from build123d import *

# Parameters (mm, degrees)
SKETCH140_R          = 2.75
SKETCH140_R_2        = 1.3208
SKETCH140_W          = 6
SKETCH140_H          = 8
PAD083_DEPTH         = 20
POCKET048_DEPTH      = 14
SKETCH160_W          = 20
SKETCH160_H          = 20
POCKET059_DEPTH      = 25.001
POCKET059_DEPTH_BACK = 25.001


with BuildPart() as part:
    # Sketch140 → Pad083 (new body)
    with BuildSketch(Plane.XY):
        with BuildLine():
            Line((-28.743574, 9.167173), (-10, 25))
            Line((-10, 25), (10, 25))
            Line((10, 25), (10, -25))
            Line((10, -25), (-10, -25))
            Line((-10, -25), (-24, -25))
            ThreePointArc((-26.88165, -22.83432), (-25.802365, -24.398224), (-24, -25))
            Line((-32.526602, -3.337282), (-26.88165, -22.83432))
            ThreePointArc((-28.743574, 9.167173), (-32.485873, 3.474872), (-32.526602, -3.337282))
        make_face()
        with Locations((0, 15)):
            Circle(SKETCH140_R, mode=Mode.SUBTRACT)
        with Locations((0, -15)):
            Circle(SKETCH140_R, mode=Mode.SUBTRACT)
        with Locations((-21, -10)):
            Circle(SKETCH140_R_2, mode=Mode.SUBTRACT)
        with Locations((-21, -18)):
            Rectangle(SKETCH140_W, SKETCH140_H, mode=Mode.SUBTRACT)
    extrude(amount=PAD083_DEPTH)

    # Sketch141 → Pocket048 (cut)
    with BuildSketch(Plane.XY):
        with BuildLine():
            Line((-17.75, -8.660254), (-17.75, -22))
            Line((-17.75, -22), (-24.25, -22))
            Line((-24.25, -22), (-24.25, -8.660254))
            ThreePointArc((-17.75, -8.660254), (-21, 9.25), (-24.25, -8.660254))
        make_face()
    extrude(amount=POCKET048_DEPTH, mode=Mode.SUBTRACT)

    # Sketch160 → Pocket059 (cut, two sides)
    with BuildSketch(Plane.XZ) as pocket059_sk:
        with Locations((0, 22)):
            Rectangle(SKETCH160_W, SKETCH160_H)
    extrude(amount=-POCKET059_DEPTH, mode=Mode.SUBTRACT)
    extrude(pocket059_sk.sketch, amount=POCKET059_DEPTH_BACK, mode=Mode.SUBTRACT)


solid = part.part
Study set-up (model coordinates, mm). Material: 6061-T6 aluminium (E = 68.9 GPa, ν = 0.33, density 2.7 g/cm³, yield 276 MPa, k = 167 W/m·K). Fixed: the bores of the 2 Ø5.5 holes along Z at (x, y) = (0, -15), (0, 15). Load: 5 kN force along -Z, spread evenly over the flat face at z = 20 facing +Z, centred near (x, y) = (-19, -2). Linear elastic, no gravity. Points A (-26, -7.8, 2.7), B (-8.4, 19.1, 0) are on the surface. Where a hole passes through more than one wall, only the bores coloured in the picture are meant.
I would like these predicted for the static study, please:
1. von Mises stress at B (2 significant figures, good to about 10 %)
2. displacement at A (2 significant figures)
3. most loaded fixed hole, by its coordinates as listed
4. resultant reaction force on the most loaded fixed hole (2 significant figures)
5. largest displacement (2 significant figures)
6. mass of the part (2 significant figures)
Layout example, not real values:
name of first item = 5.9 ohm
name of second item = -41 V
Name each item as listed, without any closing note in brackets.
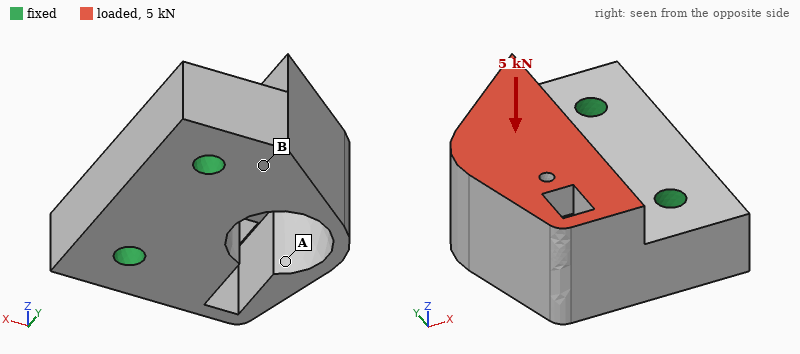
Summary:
von Mises stress at B = 58 MPa
displacement at A = 0.075 mm
most loaded fixed hole, by its coordinates as listed = (0, -15)
resultant reaction force on the most loaded fixed hole = 2.7 kN
largest displacement = 0.10 mm
mass of the part = 62 g
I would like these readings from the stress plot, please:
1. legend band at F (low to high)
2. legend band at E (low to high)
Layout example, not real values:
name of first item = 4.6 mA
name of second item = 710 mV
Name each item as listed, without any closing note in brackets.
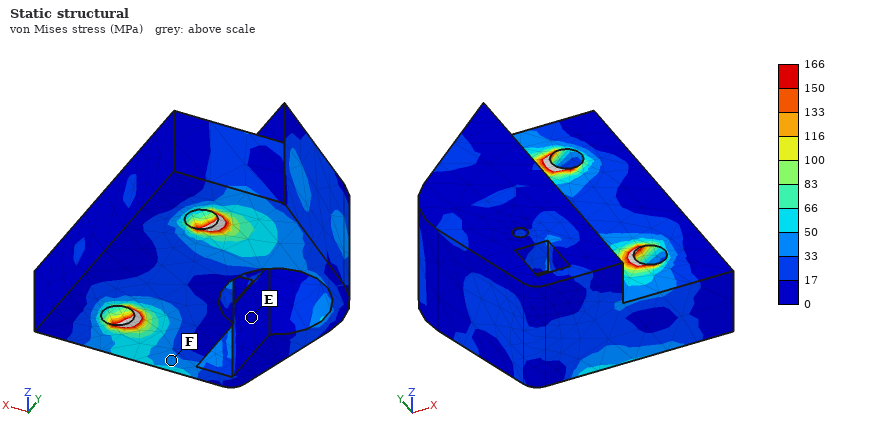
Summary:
legend band at F = 33 to 50 MPa
legend band at E = 0 to 17 MPa
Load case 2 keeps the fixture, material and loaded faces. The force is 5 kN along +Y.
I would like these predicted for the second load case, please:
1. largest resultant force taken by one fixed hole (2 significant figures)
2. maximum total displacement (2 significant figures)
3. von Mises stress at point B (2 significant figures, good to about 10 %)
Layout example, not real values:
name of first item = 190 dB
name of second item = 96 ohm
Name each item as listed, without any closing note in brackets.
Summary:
largest resultant force taken by one fixed hole = 4.1 kN
maximum total displacement = 33 µm
von Mises stress at point B = 12 MPa
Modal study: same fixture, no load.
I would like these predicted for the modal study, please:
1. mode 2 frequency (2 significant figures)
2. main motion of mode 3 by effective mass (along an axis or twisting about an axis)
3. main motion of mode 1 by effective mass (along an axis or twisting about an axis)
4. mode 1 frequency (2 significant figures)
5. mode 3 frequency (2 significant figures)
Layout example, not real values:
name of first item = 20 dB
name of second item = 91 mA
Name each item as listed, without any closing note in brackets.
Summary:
mode 2 frequency = 13 kHz
main motion of mode 3 by effective mass = along Y
main motion of mode 1 by effective mass = along Z
mode 1 frequency = 7900 Hz
mode 3 frequency = 17 kHz
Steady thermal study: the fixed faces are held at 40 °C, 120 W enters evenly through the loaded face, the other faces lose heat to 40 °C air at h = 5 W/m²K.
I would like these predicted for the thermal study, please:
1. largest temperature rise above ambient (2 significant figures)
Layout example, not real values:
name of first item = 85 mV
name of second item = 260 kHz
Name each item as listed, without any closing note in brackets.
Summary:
largest temperature rise above ambient = 48 K
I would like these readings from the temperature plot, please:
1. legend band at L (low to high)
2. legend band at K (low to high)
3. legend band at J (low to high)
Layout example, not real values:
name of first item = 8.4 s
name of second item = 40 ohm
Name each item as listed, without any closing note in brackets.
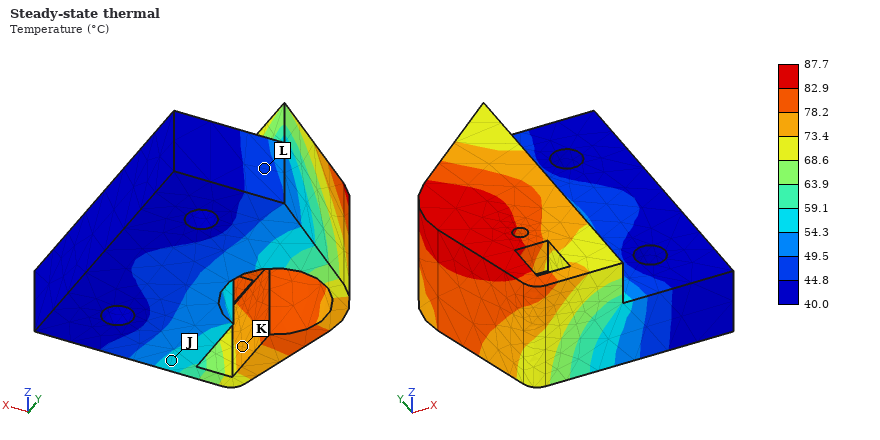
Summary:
legend band at L = 44.8 to 49.5 °C
legend band at K = 73.4 to 78.2 °C
legend band at J = 54.3 to 59.1 °C
